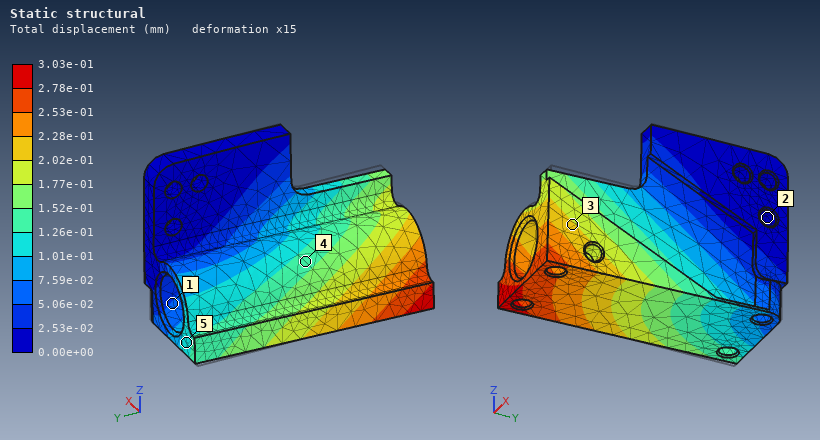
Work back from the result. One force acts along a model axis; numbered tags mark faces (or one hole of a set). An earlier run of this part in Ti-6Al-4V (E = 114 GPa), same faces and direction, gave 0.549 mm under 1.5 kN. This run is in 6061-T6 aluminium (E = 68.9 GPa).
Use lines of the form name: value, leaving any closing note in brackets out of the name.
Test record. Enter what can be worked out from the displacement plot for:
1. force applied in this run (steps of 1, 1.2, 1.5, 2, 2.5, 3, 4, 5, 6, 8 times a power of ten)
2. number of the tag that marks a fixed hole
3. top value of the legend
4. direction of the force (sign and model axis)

force applied in this run: 500 N
number of the tag that marks a fixed hole: 2
top value of the legend: 3.03e-01 mm
direction of the force: -X
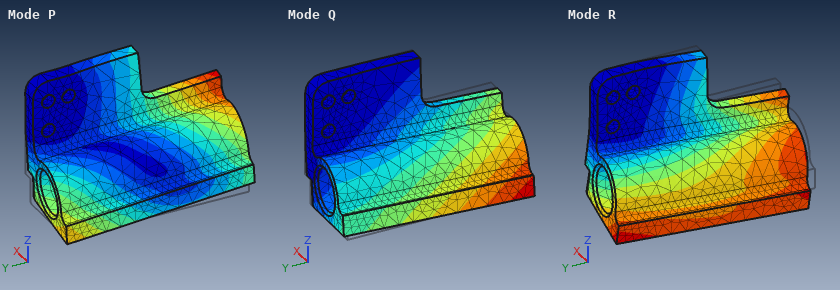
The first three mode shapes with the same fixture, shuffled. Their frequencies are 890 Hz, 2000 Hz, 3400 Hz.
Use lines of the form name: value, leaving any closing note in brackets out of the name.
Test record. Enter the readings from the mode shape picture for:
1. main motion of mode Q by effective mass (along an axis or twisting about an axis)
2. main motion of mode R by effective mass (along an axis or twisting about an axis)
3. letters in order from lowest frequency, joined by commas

main motion of mode Q by effective mass: along X
main motion of mode R by effective mass: along Z
letters in order from lowest frequency, joined by commas: Q, R, P
